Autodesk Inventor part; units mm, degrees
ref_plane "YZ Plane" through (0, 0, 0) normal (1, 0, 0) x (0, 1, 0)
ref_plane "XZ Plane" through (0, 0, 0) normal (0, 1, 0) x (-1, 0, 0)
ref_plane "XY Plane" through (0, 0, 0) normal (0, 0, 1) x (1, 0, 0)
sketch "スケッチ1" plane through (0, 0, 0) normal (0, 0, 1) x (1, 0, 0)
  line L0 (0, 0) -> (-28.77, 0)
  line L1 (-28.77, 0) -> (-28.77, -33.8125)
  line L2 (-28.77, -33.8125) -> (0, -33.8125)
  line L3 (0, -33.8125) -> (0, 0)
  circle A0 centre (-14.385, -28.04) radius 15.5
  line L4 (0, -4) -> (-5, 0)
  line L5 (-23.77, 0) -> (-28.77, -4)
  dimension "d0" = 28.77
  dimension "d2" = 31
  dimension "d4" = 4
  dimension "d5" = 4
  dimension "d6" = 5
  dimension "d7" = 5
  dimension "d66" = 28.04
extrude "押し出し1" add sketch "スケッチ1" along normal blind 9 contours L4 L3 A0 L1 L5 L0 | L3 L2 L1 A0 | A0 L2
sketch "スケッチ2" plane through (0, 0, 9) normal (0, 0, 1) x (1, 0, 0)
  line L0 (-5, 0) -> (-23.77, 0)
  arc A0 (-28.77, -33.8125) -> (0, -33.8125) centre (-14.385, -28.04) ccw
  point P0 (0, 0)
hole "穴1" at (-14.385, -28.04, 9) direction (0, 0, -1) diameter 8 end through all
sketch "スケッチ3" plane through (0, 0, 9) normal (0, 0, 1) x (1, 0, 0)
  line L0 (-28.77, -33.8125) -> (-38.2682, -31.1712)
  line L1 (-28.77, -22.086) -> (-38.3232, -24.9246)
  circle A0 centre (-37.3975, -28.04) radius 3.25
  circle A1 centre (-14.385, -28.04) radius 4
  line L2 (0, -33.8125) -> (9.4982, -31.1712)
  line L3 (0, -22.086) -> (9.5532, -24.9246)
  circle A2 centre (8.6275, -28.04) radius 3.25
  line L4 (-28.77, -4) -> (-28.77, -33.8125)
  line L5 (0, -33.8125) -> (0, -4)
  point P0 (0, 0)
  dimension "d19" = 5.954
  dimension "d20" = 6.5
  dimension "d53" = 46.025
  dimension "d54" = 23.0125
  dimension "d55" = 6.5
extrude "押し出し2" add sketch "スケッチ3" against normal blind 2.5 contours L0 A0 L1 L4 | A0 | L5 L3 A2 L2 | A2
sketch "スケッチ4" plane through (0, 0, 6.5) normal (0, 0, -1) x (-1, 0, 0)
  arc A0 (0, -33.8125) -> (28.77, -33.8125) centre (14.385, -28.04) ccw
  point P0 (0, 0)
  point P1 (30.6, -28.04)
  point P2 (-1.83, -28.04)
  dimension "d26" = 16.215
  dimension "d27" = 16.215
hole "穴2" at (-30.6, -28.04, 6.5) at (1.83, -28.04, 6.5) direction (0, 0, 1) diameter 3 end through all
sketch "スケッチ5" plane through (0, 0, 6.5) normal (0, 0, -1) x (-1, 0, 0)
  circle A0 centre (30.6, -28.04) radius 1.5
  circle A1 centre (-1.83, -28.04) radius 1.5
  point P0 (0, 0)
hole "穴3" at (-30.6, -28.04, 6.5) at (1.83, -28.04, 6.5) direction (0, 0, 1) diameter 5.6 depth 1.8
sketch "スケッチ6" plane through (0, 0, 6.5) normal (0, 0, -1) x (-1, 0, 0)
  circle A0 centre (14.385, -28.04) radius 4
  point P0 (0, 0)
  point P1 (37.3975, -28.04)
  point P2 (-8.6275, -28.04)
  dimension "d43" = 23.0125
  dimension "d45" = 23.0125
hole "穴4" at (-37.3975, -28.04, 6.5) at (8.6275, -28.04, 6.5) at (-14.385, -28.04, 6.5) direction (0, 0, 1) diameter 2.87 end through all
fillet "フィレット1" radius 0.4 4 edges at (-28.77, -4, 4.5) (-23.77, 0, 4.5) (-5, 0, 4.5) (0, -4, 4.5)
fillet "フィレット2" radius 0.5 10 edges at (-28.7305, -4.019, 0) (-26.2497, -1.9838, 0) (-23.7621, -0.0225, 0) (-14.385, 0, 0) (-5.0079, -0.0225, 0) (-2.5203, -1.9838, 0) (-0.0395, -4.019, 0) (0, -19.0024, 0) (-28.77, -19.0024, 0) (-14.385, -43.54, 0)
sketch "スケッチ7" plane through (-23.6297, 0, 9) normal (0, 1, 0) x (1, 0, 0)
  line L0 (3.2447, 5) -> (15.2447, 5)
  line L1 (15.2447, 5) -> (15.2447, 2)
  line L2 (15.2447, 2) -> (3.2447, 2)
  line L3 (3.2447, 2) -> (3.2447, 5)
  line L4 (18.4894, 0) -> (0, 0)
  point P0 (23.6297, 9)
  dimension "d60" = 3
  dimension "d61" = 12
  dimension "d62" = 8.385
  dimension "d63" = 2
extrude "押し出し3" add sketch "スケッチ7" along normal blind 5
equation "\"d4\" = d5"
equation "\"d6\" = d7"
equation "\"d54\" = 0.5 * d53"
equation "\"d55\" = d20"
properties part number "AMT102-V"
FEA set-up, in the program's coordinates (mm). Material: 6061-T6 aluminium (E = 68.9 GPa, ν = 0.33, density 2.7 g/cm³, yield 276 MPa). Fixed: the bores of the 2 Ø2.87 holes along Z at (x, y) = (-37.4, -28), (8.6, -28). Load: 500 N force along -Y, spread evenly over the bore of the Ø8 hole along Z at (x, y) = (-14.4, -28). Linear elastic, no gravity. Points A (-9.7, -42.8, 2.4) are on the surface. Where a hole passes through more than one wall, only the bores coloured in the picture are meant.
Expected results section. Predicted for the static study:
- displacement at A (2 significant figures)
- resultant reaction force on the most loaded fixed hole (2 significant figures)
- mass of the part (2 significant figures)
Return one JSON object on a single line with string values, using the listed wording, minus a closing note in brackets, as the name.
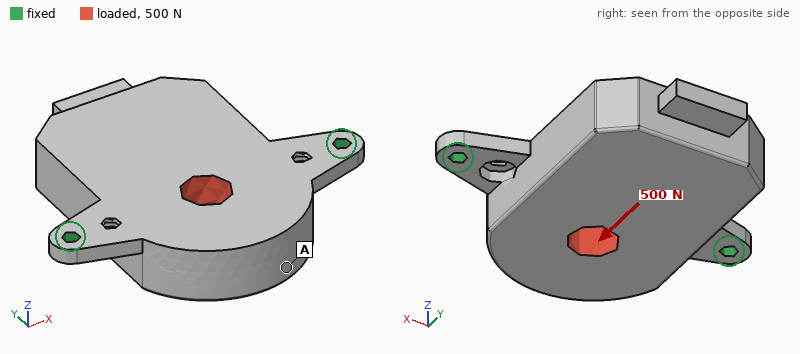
{"displacement at A": "0.11 mm", "resultant reaction force on the most loaded fixed hole": "250 N", "mass of the part": "28 g"}
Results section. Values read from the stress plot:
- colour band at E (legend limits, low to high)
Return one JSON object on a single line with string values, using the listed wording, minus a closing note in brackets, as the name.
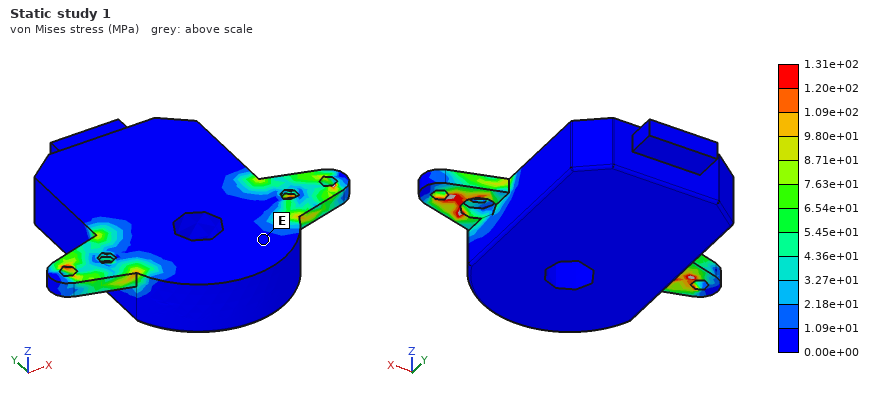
{"colour band at E": "0.00e+00 to 1.09e+01 MPa"}
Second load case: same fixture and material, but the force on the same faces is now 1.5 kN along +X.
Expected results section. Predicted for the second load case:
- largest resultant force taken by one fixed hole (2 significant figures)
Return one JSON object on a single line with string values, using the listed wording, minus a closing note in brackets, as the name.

{"largest resultant force taken by one fixed hole": "760 N"}
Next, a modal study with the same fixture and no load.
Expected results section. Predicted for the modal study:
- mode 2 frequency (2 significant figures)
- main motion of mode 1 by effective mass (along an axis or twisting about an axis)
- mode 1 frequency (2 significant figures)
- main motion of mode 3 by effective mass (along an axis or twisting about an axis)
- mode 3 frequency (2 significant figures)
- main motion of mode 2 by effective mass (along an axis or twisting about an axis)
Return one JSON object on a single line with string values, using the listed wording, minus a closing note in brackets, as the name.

{"mode 2 frequency": "4300 Hz", "main motion of mode 1 by effective mass": "along Z", "mode 1 frequency": "1000 Hz", "main motion of mode 3 by effective mass": "along X", "mode 3 frequency": "6900 Hz", "main motion of mode 2 by effective mass": "along Z"}
